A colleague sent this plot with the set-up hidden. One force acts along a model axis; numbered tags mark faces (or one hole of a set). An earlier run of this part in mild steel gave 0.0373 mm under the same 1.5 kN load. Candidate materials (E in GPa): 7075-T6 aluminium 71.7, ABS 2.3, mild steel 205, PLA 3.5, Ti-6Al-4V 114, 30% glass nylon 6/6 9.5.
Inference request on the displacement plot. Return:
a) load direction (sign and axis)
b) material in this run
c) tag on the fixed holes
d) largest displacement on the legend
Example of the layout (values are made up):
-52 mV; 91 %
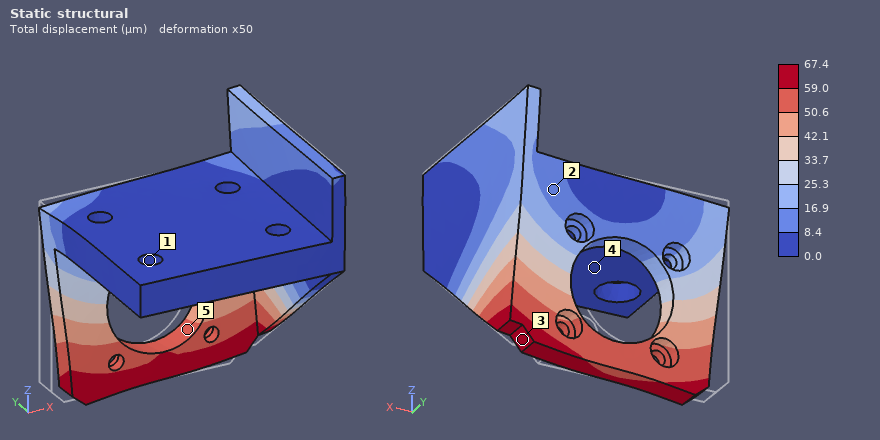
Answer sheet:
+X; Ti-6Al-4V; 1; 67.4 µm
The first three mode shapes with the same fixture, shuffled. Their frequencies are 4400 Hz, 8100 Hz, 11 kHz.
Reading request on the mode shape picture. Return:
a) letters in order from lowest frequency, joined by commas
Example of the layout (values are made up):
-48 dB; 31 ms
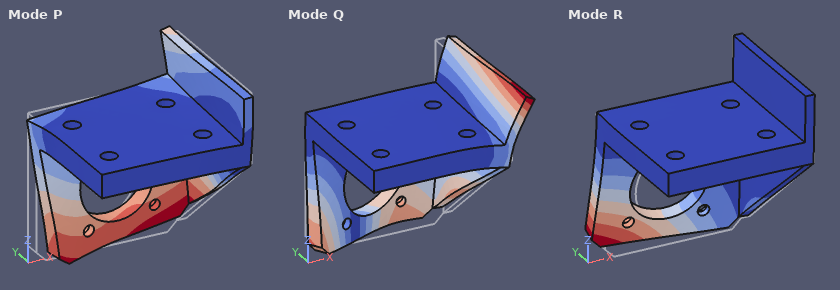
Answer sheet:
R, P, Q
